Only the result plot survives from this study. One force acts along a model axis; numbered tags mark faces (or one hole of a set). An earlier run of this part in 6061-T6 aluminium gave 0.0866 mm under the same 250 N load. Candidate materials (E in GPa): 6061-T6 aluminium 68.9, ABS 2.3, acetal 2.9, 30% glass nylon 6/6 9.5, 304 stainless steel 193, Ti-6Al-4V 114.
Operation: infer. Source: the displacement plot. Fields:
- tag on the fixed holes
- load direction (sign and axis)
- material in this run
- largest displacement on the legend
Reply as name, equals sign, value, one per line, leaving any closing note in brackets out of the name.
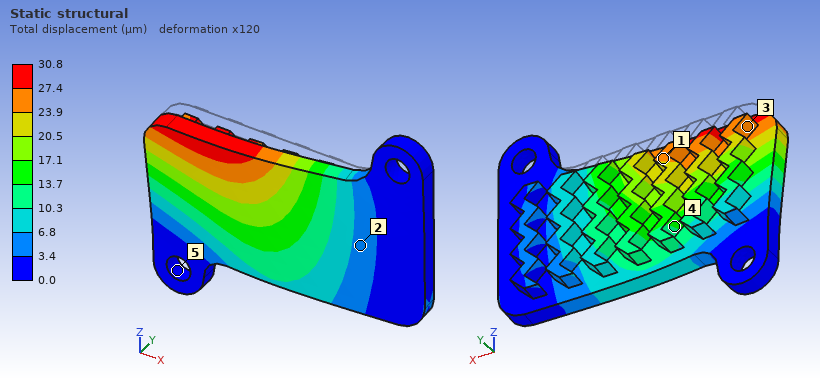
tag on the fixed holes = 5
load direction = -Y
material in this run = 304 stainless steel
largest displacement on the legend = 30.8 µm
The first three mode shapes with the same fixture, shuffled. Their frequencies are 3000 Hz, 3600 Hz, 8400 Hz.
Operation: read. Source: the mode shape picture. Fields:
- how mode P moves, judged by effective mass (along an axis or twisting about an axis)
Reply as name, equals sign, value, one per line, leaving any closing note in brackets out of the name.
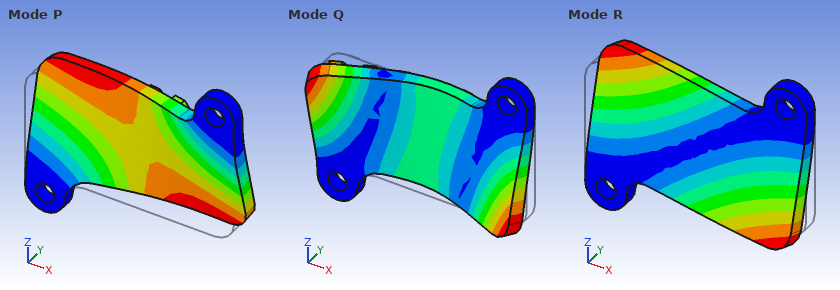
how mode P moves, judged by effective mass = along Y
